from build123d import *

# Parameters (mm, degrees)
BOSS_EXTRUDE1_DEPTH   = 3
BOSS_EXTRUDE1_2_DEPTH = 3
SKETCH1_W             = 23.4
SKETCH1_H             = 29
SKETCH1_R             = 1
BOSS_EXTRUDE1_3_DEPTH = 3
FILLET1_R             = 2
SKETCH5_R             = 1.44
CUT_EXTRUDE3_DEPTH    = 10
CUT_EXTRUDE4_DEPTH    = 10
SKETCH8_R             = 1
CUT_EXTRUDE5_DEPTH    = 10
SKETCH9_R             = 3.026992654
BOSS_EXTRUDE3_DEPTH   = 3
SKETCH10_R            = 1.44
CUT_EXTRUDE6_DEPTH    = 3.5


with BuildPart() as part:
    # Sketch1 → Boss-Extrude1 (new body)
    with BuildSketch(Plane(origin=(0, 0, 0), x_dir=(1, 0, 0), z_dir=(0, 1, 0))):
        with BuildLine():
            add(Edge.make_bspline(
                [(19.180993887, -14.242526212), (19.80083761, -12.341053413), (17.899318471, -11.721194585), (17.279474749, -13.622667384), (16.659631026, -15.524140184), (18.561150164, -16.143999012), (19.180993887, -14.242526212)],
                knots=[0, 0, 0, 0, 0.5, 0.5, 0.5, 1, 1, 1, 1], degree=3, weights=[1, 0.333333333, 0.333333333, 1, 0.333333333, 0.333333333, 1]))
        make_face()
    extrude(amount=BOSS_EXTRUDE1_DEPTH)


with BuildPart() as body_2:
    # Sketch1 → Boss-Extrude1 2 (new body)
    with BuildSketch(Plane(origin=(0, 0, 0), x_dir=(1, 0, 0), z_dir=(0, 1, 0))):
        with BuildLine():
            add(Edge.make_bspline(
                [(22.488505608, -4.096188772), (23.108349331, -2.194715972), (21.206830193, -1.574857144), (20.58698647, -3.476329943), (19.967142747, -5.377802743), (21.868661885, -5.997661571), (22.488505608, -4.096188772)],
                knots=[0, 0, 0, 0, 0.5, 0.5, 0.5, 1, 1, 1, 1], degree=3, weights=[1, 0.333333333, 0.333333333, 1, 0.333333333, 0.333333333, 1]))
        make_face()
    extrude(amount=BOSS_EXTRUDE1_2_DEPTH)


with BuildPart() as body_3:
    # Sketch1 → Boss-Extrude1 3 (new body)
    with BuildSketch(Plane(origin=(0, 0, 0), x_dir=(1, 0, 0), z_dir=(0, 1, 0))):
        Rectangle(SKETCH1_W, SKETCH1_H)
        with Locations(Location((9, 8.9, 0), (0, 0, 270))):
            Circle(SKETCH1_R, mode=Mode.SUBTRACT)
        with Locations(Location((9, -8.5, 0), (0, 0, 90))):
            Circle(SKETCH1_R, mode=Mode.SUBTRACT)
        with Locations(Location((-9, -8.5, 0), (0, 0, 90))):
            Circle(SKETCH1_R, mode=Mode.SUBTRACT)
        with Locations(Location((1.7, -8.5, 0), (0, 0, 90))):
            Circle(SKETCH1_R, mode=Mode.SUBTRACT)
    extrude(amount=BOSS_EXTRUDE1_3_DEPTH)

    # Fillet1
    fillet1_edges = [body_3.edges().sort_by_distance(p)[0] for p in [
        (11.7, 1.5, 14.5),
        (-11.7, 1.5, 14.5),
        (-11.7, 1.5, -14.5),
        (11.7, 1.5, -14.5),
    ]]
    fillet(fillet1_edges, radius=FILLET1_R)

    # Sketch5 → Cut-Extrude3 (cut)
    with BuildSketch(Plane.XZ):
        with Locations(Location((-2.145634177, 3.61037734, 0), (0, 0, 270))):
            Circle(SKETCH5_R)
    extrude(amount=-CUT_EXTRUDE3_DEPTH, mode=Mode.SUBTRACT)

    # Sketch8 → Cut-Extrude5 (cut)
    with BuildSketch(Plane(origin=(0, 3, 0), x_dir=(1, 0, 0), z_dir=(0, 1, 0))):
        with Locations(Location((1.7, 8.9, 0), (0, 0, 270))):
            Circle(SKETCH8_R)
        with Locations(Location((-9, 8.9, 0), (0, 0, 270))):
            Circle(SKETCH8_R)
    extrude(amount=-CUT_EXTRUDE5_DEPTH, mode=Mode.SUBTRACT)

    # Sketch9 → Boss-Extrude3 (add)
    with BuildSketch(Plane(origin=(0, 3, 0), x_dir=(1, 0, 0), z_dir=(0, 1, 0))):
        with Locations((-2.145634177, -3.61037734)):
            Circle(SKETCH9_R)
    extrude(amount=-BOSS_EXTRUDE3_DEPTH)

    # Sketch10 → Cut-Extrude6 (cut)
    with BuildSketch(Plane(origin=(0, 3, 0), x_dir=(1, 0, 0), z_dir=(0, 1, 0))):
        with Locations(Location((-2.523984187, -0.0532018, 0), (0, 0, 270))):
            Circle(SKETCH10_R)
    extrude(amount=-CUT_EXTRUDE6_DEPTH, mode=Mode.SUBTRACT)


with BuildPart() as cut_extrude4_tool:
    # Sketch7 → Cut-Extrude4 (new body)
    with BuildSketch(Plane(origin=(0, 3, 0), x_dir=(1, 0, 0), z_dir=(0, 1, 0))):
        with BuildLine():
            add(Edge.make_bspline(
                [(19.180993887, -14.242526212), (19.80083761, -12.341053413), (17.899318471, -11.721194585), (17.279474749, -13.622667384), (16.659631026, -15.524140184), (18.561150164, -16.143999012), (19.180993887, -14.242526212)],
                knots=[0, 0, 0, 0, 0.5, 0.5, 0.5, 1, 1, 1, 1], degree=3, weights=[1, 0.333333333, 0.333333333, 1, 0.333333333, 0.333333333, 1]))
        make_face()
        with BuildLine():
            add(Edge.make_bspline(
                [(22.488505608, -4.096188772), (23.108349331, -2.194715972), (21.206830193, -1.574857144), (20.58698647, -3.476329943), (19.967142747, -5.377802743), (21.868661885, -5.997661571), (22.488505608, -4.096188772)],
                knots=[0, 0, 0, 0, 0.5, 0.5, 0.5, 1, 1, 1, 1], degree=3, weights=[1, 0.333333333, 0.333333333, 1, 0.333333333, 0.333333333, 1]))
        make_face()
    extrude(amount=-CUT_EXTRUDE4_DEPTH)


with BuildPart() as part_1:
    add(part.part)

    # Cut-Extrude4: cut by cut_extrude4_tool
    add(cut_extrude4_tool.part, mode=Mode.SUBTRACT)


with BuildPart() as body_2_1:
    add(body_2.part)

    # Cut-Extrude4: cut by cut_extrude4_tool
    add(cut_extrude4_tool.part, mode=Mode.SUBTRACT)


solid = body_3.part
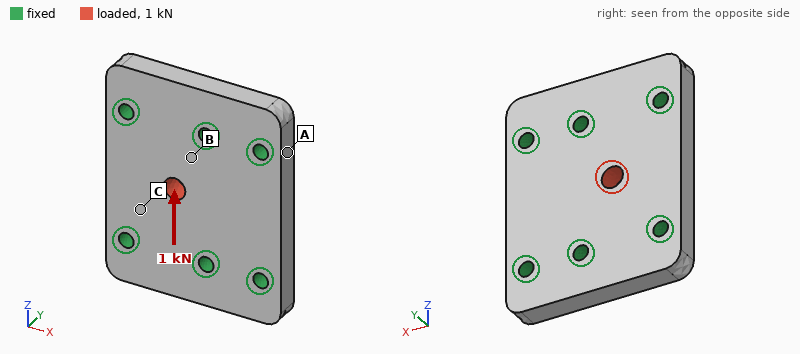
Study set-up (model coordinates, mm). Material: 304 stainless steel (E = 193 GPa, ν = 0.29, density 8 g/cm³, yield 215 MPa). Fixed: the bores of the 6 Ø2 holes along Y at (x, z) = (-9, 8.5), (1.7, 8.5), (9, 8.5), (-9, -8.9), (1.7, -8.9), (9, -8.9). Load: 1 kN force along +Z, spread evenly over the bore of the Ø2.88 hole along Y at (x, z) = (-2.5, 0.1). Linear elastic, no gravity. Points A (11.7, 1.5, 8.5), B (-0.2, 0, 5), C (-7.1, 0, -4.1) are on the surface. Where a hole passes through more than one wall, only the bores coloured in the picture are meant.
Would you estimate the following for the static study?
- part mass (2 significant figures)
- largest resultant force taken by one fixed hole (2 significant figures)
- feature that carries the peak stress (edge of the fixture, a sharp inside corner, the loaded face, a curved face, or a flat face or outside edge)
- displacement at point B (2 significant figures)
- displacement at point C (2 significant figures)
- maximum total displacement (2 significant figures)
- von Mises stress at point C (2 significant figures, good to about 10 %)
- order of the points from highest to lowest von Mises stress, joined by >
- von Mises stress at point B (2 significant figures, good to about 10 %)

16 g
260 N
the loaded face
0.34 µm
0.30 µm
0.98 µm
12 MPa
B > C > A
20 MPa
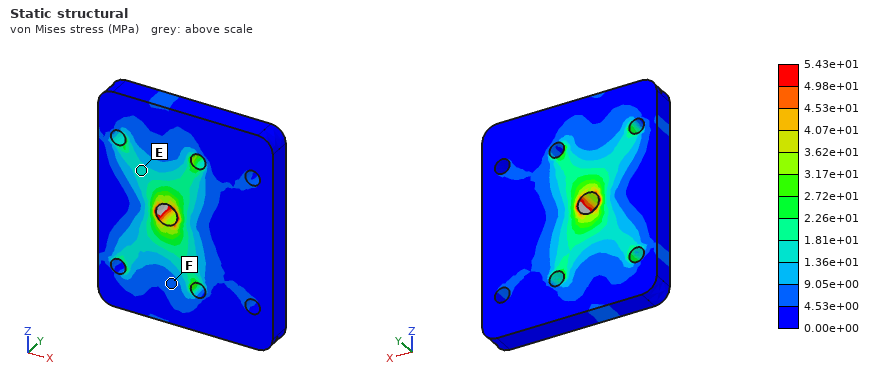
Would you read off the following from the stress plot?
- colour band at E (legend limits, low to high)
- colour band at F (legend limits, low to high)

1.36e+01 to 1.81e+01 MPa
4.53e+00 to 9.05e+00 MPa
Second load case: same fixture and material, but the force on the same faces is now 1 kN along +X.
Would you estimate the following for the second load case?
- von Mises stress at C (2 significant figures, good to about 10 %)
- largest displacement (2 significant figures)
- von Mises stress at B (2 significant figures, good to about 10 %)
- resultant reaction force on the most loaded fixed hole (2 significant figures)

17 MPa
1.4 µm
17 MPa
230 N
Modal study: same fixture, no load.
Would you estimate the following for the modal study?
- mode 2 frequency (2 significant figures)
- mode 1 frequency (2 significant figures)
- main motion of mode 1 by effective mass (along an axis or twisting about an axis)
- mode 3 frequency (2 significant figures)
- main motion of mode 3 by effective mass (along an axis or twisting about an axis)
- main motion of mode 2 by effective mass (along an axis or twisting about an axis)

48 kHz
41 kHz
along Y
55 kHz
along Y
twisting about Z
